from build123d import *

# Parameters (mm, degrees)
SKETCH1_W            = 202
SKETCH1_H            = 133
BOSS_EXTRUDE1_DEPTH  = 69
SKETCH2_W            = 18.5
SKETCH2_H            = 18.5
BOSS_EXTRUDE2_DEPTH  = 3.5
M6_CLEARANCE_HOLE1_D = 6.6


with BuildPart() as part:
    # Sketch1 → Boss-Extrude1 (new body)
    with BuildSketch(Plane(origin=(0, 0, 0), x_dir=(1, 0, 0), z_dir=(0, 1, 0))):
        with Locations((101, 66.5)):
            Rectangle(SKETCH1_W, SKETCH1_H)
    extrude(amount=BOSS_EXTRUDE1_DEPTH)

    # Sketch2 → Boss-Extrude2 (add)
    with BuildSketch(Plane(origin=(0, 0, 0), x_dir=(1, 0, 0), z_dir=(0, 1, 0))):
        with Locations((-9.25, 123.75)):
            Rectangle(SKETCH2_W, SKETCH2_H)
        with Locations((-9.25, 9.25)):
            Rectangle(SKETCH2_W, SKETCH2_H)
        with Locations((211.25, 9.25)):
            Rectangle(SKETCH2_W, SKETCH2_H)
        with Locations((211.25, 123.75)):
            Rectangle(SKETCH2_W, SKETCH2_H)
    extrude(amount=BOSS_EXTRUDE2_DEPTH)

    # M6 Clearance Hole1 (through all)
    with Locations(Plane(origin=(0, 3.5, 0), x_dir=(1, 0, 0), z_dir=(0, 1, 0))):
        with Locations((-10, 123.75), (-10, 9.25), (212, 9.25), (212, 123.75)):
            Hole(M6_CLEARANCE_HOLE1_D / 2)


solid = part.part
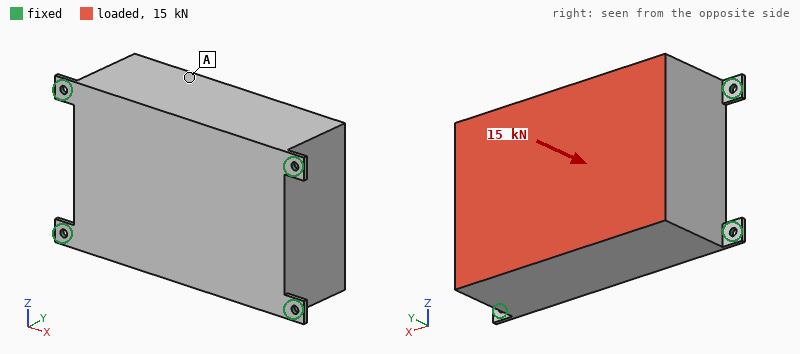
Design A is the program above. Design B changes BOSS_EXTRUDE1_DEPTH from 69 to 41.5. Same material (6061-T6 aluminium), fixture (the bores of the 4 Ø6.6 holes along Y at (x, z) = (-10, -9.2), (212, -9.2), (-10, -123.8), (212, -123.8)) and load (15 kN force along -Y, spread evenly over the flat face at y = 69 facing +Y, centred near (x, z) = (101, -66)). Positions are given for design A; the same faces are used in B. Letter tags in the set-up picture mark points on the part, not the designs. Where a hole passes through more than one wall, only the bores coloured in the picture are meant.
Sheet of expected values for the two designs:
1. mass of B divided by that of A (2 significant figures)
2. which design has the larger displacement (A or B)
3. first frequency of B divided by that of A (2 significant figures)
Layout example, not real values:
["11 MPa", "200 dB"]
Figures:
["0.60", "B", "1.3"]
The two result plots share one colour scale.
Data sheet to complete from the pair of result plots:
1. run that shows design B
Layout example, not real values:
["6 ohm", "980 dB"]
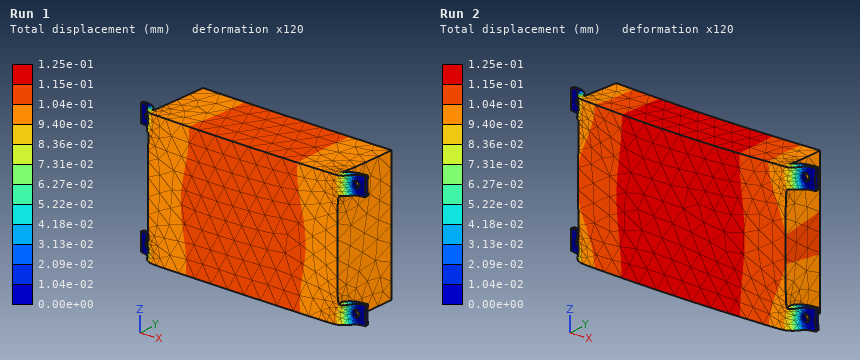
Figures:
["Run 2"]
